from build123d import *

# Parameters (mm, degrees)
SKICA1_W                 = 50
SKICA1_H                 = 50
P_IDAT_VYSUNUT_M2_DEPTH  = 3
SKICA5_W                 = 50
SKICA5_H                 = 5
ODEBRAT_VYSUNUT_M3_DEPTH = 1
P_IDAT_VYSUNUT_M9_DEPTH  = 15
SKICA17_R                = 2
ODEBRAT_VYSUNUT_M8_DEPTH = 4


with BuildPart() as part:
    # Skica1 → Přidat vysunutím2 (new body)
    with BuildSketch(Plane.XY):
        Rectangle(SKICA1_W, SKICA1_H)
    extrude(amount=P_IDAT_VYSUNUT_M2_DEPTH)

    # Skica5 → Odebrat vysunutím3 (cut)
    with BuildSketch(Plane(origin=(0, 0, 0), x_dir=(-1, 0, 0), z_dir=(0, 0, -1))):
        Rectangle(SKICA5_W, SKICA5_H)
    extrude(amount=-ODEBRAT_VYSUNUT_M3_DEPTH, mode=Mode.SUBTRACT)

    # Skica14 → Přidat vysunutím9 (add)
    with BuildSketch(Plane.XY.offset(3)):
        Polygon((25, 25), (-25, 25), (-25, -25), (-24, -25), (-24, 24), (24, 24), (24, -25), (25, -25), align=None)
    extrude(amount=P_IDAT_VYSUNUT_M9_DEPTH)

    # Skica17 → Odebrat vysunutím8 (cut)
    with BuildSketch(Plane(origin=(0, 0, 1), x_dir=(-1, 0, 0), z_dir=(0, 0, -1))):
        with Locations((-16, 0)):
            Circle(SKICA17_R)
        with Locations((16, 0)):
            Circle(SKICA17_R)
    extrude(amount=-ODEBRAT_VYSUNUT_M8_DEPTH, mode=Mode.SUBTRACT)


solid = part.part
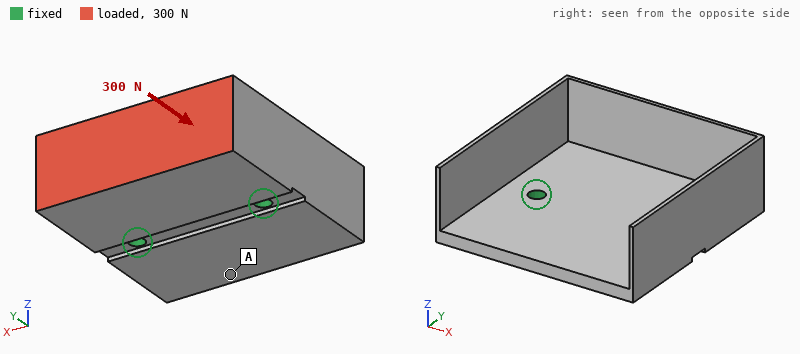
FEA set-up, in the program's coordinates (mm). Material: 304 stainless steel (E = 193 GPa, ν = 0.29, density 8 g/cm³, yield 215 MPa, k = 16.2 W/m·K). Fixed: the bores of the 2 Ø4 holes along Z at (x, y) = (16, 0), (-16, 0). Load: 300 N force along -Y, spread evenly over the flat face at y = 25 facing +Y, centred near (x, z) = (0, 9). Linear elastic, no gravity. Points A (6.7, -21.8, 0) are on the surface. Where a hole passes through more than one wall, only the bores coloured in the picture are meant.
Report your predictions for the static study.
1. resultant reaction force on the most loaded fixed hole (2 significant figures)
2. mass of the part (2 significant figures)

150 N
75 g
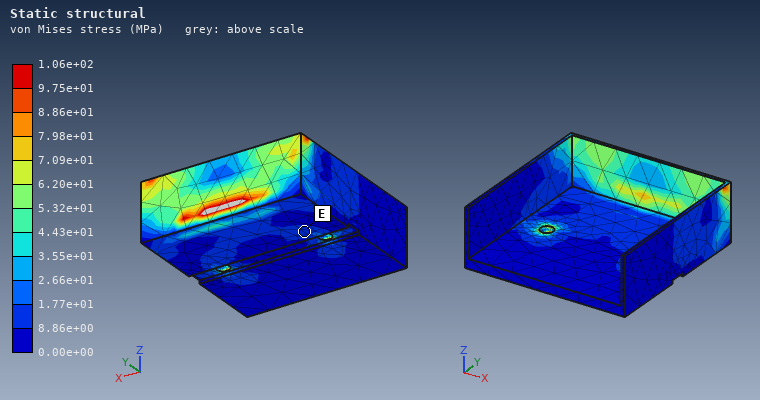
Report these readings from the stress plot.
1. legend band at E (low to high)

8.86e+00 to 1.77e+01 MPa
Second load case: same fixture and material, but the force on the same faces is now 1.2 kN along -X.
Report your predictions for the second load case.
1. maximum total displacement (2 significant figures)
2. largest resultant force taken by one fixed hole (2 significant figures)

95 µm
1.1 kN
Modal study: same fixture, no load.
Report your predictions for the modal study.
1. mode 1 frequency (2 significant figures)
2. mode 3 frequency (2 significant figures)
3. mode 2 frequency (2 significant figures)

2100 Hz
3600 Hz
3100 Hz
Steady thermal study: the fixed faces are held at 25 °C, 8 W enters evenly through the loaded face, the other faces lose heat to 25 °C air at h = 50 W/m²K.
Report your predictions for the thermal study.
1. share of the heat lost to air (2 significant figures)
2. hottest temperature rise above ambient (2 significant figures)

76 %
69 K
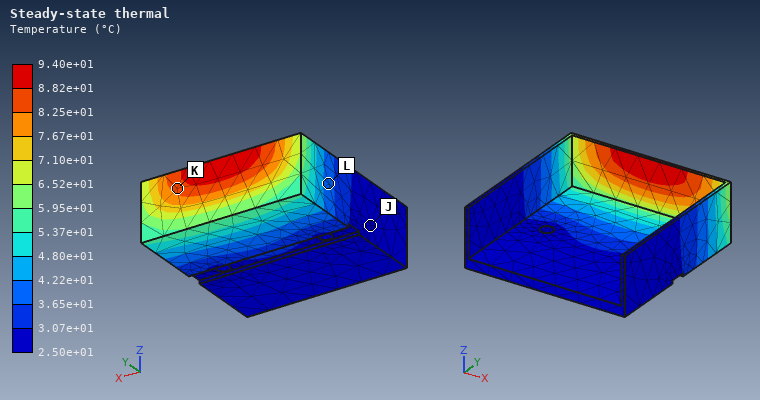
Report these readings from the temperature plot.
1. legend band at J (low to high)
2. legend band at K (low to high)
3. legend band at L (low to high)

2.50e+01 to 3.07e+01 °C
8.25e+01 to 8.82e+01 °C
3.65e+01 to 4.22e+01 °C
